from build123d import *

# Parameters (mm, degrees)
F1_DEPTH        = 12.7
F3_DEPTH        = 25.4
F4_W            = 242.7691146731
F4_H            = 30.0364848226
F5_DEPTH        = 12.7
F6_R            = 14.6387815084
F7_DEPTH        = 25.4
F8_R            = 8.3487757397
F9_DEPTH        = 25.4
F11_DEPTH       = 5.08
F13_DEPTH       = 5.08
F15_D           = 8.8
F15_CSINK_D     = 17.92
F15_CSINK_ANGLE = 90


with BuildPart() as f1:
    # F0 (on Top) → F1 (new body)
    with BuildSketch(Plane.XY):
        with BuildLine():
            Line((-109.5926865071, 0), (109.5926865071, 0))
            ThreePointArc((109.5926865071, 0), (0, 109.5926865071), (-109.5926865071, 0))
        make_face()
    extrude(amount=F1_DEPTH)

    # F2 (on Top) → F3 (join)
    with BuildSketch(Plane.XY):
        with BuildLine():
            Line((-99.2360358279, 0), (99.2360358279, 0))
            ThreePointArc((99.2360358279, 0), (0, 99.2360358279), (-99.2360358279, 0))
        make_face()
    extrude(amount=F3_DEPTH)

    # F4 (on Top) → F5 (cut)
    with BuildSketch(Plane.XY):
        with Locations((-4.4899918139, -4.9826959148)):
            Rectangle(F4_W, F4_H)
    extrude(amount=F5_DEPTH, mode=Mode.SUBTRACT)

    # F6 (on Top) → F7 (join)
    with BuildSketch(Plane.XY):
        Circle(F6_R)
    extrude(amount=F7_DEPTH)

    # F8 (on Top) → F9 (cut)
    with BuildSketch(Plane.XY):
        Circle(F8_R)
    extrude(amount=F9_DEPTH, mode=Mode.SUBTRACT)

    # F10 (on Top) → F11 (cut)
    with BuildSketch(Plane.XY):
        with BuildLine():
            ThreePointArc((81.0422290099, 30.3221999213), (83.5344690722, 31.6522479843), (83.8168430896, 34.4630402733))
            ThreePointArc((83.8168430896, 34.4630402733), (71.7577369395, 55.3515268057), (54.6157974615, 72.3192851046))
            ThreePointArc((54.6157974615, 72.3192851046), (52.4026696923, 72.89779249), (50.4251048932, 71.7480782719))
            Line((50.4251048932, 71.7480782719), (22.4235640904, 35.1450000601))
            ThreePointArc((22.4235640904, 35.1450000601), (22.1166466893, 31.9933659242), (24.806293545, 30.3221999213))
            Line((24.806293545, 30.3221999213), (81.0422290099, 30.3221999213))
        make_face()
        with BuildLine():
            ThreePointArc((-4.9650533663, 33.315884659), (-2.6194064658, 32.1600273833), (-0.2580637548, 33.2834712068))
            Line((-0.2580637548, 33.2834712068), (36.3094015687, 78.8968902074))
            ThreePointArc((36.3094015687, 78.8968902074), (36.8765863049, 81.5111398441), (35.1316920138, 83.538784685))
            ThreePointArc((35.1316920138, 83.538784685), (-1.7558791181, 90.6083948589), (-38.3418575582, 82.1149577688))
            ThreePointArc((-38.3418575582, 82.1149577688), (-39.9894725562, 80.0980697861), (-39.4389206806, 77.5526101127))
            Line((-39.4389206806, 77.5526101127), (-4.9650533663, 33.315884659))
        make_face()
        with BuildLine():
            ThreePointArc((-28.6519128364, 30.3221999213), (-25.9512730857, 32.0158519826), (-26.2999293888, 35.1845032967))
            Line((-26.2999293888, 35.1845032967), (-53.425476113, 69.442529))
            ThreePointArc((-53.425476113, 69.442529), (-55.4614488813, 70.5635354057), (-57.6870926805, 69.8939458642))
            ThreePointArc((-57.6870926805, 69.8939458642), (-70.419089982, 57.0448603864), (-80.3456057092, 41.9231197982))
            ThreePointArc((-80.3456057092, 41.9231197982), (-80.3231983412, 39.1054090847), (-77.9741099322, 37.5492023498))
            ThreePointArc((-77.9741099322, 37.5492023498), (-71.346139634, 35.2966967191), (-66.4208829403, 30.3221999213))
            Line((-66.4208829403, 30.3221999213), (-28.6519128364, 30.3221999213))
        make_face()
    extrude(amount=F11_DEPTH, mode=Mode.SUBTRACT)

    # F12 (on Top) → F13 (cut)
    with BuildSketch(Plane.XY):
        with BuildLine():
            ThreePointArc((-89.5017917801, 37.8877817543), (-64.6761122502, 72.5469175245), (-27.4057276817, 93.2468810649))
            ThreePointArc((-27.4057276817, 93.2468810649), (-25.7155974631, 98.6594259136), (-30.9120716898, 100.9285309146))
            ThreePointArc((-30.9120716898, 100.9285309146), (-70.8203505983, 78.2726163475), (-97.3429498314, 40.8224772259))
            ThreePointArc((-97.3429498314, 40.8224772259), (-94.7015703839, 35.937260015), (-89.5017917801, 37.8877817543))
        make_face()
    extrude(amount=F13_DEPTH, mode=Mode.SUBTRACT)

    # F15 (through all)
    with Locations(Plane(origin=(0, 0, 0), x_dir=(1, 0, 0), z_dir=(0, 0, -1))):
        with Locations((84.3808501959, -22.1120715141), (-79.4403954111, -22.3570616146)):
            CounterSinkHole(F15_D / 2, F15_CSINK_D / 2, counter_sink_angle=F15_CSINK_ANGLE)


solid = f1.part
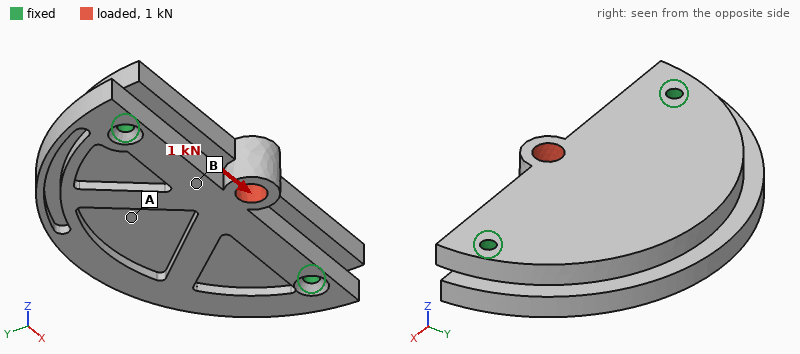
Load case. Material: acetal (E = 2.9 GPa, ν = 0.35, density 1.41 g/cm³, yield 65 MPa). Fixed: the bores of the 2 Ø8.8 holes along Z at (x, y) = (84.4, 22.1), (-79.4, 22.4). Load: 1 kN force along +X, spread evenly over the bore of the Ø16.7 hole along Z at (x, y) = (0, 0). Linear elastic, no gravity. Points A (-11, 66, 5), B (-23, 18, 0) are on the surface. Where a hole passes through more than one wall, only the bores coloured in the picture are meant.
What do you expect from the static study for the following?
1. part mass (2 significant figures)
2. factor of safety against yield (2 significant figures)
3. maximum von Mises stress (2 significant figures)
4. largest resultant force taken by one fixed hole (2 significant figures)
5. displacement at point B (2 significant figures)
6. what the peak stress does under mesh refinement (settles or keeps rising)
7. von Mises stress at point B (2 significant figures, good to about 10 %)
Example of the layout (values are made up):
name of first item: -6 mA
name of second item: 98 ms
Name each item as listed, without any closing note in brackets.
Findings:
part mass: 530 g
factor of safety against yield: 8.9
maximum von Mises stress: 7.3 MPa
largest resultant force taken by one fixed hole: 540 N
displacement at point B: 15 µm
what the peak stress does under mesh refinement: settles
von Mises stress at point B: 0.97 MPa
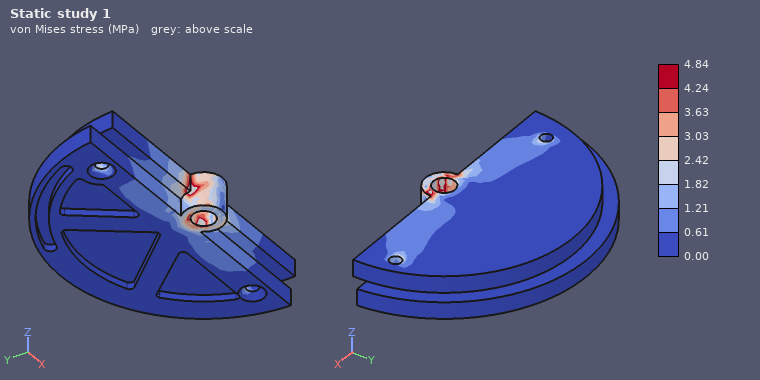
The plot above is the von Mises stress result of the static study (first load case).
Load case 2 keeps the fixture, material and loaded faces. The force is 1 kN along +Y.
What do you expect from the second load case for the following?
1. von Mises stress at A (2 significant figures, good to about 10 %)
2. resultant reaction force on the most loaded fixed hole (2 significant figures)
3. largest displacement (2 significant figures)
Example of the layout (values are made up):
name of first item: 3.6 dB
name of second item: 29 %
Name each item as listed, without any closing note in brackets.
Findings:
von Mises stress at A: 0.60 MPa
resultant reaction force on the most loaded fixed hole: 560 N
largest displacement: 82 µm
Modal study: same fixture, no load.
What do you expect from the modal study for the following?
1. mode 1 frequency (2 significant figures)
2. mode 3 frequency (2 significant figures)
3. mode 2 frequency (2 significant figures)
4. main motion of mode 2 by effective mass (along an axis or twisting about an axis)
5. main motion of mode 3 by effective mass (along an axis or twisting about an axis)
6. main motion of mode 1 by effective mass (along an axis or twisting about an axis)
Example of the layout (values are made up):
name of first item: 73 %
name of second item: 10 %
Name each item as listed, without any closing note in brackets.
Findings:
mode 1 frequency: 490 Hz
mode 3 frequency: 1300 Hz
mode 2 frequency: 1000 Hz
main motion of mode 2 by effective mass: along Z
main motion of mode 3 by effective mass: twisting about Y
main motion of mode 1 by effective mass: along Z
